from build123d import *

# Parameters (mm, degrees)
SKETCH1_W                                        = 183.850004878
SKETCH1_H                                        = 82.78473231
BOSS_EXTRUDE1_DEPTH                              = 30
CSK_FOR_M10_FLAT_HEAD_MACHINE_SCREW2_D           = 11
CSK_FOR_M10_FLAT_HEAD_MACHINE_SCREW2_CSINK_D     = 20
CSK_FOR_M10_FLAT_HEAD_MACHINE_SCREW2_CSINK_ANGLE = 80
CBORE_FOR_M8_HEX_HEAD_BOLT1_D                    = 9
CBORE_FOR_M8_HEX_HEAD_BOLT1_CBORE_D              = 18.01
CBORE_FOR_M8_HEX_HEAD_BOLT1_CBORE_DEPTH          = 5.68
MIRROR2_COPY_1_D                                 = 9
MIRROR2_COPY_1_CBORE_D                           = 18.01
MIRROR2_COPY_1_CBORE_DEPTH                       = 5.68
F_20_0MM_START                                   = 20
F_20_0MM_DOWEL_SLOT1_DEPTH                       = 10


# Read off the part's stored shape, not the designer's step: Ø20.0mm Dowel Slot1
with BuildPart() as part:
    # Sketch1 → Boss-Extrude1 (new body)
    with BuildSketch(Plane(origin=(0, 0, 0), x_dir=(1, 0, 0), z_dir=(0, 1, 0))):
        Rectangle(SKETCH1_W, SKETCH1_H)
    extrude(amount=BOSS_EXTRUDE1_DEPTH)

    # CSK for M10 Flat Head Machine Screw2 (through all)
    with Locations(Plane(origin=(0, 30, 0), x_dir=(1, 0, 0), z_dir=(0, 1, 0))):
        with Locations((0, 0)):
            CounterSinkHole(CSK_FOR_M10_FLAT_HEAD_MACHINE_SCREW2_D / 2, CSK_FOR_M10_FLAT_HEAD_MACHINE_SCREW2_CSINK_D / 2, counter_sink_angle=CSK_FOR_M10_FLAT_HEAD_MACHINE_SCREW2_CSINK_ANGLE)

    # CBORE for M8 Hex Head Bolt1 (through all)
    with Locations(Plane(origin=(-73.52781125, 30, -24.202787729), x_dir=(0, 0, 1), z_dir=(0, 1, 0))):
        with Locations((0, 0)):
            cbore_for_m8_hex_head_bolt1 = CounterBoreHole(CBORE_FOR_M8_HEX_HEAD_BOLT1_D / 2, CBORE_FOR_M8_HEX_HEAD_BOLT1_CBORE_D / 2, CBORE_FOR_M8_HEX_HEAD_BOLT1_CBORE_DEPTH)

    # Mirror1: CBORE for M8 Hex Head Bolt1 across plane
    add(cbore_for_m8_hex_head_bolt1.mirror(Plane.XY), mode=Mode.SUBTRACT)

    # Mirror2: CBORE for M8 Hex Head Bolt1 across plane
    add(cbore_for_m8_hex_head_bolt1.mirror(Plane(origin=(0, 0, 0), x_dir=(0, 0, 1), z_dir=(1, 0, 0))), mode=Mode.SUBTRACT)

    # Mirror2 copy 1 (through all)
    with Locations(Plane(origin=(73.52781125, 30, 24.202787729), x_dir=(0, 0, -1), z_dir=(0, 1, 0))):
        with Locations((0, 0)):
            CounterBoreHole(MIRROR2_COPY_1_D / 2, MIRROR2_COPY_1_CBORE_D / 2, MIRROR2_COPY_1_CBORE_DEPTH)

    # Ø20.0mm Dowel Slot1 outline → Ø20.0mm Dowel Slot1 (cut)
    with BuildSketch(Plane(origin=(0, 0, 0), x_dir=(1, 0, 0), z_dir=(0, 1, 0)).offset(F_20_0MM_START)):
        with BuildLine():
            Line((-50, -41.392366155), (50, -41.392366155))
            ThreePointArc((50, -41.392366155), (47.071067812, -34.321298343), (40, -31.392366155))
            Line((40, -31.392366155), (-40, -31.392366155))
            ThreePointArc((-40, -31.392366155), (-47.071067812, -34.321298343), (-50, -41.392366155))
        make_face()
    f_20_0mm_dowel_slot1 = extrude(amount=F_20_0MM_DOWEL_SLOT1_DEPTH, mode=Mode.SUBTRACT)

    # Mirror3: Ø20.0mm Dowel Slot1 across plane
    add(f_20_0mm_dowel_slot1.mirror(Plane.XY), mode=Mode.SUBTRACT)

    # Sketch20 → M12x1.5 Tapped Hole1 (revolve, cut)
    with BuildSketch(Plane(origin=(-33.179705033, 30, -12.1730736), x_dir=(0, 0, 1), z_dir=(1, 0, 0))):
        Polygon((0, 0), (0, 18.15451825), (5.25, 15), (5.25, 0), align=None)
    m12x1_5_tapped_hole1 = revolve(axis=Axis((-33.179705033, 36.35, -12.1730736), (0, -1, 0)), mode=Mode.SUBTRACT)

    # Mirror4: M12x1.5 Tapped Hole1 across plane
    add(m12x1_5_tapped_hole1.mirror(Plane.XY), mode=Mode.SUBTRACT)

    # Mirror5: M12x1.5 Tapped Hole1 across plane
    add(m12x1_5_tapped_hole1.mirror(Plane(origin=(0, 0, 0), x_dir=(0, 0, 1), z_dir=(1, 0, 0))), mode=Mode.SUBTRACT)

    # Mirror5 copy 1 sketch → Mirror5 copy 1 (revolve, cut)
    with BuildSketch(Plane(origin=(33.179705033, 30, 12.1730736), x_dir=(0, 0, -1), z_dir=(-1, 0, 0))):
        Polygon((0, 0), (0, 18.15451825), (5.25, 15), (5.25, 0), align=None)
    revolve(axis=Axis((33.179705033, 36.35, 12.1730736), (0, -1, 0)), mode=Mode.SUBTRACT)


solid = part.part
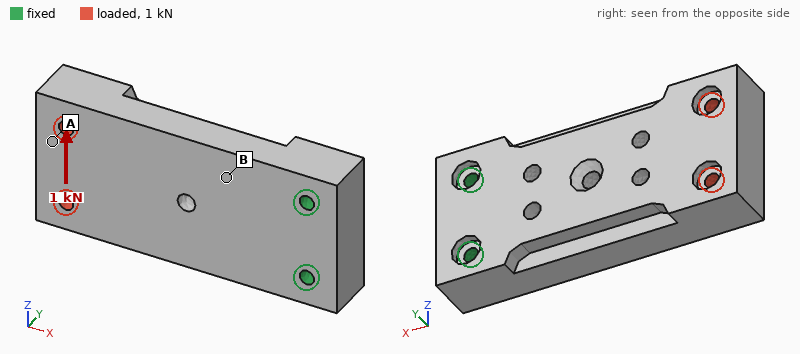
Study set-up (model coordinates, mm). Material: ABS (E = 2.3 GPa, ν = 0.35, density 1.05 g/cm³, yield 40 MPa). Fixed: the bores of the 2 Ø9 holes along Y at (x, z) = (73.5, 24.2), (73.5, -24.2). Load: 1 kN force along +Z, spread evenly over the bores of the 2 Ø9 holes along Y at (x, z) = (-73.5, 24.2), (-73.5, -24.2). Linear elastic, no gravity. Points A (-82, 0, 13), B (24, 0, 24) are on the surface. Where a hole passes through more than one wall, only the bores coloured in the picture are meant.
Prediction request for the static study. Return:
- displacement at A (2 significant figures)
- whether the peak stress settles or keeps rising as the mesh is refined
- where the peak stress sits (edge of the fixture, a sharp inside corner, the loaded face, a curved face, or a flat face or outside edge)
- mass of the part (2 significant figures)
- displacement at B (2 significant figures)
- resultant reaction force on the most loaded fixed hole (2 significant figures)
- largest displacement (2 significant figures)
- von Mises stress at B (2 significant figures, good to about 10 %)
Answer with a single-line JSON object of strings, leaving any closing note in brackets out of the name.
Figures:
{"displacement at A": "0.60 mm", "whether the peak stress settles or keeps rising as the mesh is refined": "keeps rising", "where the peak stress sits": "edge of the fixture", "mass of the part": "440 g", "displacement at B": "0.13 mm", "resultant reaction force on the most loaded fixed hole": "2.8 kN", "largest displacement": "0.67 mm", "von Mises stress at B": "2.2 MPa"}
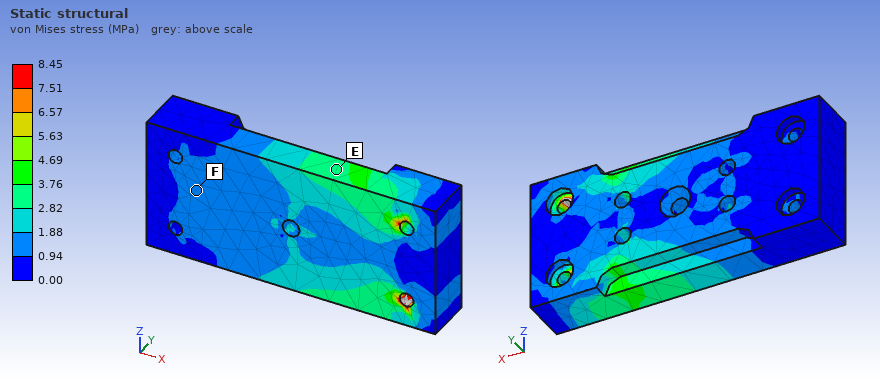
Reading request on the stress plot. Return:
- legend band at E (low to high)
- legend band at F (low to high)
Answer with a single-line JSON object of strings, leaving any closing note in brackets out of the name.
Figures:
{"legend band at E": "2.82 to 3.76 MPa", "legend band at F": "0.94 to 1.88 MPa"}
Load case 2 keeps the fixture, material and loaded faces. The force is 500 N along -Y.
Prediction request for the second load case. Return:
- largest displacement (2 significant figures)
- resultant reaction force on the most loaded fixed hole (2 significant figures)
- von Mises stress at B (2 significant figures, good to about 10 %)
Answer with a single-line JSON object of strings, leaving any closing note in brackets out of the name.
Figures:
{"largest displacement": "2.1 mm", "resultant reaction force on the most loaded fixed hole": "250 N", "von Mises stress at B": "4.6 MPa"}
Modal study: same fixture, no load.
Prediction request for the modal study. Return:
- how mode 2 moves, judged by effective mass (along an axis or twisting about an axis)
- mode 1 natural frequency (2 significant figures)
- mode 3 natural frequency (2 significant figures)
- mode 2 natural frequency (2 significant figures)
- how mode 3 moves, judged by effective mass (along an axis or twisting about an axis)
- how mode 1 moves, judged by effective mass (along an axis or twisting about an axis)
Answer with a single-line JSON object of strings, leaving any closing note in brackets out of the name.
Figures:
{"how mode 2 moves, judged by effective mass": "along Z", "mode 1 natural frequency": "220 Hz", "mode 3 natural frequency": "820 Hz", "mode 2 natural frequency": "550 Hz", "how mode 3 moves, judged by effective mass": "twisting about X", "how mode 1 moves, judged by effective mass": "along Y"}
